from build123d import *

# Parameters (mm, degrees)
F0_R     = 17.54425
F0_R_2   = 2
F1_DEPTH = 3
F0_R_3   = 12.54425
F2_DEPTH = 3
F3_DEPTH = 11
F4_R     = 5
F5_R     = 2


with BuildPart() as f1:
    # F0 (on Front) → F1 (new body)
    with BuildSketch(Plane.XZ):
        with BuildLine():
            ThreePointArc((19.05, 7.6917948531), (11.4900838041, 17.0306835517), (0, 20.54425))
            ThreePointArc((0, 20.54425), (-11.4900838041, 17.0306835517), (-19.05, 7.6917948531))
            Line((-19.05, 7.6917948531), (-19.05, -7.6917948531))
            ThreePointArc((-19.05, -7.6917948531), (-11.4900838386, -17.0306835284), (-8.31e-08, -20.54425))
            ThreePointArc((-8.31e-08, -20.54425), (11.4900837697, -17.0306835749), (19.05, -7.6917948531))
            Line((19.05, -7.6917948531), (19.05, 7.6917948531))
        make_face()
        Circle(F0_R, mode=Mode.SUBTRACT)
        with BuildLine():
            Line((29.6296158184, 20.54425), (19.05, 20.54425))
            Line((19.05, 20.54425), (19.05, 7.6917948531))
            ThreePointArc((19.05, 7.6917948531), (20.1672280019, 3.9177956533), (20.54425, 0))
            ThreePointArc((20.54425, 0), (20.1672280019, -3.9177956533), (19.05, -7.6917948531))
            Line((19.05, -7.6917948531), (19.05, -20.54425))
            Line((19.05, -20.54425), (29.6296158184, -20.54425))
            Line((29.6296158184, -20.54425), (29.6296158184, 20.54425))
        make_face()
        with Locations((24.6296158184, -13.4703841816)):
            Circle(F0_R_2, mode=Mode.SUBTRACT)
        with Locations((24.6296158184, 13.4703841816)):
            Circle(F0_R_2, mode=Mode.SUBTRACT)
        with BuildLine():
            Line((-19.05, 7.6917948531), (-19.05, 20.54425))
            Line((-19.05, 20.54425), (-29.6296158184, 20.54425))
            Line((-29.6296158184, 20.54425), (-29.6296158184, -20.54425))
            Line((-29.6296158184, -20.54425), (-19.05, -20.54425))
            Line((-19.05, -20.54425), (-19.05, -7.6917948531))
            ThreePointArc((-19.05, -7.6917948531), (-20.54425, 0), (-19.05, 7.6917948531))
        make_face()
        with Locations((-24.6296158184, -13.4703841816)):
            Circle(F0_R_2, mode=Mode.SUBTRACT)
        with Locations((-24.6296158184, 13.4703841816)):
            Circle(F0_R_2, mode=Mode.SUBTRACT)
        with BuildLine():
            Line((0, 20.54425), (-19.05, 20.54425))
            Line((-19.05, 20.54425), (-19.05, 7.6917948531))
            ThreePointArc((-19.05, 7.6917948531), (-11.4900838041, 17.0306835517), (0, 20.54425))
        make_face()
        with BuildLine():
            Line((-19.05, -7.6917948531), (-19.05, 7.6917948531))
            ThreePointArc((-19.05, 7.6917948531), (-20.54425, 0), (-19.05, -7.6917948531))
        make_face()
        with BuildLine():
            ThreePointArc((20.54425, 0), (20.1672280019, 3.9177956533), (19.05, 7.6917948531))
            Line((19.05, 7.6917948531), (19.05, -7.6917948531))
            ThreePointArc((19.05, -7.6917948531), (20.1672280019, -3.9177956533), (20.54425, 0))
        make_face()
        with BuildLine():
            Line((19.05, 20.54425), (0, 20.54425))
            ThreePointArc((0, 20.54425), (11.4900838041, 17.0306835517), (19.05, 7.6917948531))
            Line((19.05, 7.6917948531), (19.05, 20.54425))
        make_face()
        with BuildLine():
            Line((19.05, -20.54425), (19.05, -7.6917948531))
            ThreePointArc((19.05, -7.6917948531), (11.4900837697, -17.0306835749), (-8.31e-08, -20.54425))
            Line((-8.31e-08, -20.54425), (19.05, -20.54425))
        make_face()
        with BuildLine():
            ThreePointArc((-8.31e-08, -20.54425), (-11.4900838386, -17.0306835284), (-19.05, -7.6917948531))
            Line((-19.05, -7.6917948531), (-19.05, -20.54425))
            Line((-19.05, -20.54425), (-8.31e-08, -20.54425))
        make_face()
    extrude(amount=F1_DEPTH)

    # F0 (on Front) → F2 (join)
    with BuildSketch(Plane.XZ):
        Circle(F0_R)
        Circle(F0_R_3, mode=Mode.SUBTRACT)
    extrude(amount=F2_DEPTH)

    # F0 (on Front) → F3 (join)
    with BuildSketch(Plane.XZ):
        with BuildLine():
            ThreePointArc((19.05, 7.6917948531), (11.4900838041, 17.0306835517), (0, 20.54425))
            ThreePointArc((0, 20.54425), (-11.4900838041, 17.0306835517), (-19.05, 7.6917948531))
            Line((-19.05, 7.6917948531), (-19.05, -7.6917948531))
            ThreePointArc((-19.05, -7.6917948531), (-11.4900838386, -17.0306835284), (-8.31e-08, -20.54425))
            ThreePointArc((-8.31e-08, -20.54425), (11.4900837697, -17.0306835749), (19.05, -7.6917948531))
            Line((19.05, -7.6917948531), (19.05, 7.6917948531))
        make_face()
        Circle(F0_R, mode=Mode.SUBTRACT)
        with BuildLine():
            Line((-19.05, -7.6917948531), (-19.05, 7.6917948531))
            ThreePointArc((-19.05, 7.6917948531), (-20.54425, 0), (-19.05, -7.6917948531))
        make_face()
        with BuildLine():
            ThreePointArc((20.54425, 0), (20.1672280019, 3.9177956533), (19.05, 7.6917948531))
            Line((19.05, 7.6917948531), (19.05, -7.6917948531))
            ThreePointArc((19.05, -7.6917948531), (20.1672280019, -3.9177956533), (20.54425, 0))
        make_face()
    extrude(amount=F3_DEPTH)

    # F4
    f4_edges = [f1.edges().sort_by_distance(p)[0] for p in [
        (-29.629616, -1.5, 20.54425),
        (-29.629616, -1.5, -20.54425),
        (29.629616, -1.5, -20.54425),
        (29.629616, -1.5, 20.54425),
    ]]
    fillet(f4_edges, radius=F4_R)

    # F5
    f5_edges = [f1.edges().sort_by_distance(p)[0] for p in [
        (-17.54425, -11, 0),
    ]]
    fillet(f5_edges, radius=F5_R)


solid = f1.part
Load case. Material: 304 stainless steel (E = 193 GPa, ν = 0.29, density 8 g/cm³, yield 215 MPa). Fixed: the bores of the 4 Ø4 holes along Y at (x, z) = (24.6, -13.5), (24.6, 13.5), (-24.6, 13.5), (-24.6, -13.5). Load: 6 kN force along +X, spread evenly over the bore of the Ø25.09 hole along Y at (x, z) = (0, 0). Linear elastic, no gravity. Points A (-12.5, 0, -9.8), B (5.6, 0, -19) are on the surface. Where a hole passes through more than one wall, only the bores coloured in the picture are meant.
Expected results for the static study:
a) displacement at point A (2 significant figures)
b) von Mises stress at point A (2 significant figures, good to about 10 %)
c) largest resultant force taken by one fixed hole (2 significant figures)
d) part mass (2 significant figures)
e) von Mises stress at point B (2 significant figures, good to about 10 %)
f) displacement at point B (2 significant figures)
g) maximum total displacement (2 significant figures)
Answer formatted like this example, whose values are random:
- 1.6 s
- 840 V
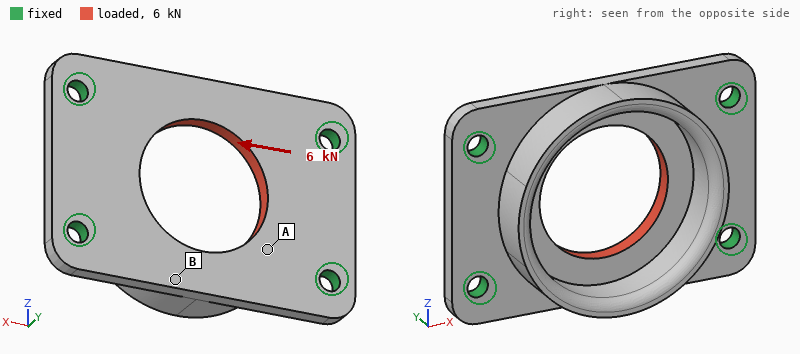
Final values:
- 2.4 µm
- 32 MPa
- 1.5 kN
- 67 g
- 9.6 MPa
- 2.3 µm
- 3.6 µm
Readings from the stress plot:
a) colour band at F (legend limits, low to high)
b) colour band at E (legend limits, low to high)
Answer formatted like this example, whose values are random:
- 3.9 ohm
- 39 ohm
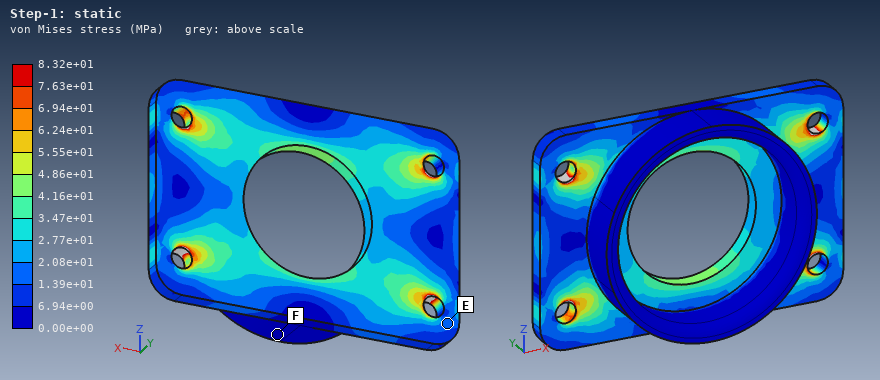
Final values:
- 0.00e+00 to 6.94e+00 MPa
- 1.39e+01 to 2.08e+01 MPa
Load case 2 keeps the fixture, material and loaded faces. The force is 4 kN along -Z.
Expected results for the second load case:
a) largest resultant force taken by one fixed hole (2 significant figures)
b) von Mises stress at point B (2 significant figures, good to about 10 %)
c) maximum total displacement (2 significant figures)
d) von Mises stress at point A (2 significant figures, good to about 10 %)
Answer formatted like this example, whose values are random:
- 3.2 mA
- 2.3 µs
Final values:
- 1.1 kN
- 29 MPa
- 8.2 µm
- 30 MPa
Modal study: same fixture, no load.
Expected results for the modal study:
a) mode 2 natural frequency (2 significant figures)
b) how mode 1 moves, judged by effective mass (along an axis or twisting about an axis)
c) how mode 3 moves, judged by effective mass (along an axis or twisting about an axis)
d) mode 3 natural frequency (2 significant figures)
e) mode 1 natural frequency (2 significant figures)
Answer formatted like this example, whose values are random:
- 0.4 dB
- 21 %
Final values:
- 8700 Hz
- along Y
- twisting about Z
- 17 kHz
- 8000 Hz
